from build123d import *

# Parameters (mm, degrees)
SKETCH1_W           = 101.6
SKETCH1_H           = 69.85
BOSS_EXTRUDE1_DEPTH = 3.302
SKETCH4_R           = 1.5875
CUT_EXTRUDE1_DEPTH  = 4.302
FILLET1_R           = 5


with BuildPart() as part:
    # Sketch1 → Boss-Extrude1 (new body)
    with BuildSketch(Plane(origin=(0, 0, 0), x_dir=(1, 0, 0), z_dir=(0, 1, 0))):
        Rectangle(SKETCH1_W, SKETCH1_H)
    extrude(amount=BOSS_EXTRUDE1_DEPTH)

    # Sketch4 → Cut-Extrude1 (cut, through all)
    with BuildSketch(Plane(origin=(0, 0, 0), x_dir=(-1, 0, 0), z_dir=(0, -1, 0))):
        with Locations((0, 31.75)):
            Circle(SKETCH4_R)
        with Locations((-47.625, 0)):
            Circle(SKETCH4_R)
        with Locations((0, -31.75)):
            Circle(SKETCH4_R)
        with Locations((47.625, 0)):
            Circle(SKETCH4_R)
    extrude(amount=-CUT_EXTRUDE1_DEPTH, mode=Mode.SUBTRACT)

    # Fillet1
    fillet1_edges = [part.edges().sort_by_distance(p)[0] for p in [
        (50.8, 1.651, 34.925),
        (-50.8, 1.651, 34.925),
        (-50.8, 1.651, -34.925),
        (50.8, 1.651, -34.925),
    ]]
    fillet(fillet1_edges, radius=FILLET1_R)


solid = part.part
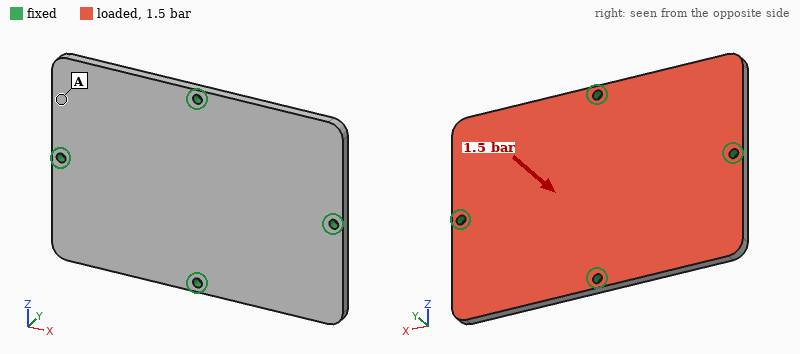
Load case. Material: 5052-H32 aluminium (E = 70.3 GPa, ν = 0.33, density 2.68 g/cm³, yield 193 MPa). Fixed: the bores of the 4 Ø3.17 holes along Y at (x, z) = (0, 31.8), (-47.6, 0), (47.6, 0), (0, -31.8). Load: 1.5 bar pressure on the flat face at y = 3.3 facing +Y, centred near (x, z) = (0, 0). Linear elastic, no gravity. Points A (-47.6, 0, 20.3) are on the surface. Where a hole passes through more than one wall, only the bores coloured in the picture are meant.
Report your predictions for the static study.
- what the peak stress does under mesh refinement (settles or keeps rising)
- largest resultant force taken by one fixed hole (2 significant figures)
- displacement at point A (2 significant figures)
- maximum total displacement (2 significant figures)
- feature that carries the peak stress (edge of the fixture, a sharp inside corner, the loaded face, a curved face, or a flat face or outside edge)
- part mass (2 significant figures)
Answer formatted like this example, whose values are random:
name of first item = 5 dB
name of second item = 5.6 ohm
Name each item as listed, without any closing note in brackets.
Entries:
what the peak stress does under mesh refinement = keeps rising
largest resultant force taken by one fixed hole = 270 N
displacement at point A = 32 µm
maximum total displacement = 62 µm
feature that carries the peak stress = edge of the fixture
part mass = 62 g
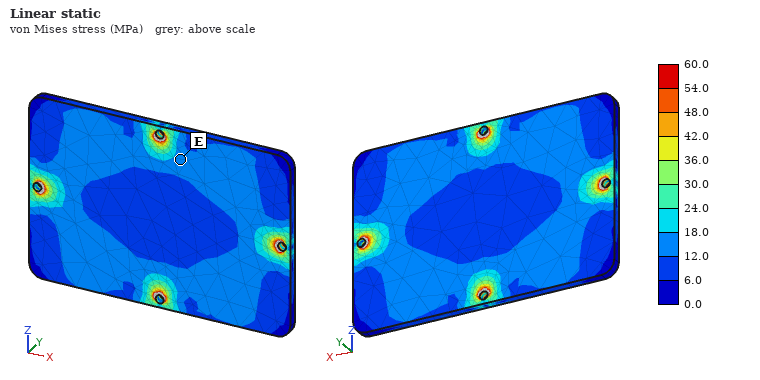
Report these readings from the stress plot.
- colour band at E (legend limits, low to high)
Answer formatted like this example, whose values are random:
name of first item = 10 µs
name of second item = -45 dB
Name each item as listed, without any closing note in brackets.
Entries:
colour band at E = 12.0 to 18.0 MPa
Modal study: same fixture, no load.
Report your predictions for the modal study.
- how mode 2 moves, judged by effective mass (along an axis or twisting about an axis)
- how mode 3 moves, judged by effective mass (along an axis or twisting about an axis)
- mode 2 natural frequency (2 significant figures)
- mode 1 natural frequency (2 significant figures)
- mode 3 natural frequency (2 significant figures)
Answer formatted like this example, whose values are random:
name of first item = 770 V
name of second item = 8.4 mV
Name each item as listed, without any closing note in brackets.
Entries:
how mode 2 moves, judged by effective mass = twisting about X
how mode 3 moves, judged by effective mass = twisting about Z
mode 2 natural frequency = 3000 Hz
mode 1 natural frequency = 2900 Hz
mode 3 natural frequency = 3200 Hz
